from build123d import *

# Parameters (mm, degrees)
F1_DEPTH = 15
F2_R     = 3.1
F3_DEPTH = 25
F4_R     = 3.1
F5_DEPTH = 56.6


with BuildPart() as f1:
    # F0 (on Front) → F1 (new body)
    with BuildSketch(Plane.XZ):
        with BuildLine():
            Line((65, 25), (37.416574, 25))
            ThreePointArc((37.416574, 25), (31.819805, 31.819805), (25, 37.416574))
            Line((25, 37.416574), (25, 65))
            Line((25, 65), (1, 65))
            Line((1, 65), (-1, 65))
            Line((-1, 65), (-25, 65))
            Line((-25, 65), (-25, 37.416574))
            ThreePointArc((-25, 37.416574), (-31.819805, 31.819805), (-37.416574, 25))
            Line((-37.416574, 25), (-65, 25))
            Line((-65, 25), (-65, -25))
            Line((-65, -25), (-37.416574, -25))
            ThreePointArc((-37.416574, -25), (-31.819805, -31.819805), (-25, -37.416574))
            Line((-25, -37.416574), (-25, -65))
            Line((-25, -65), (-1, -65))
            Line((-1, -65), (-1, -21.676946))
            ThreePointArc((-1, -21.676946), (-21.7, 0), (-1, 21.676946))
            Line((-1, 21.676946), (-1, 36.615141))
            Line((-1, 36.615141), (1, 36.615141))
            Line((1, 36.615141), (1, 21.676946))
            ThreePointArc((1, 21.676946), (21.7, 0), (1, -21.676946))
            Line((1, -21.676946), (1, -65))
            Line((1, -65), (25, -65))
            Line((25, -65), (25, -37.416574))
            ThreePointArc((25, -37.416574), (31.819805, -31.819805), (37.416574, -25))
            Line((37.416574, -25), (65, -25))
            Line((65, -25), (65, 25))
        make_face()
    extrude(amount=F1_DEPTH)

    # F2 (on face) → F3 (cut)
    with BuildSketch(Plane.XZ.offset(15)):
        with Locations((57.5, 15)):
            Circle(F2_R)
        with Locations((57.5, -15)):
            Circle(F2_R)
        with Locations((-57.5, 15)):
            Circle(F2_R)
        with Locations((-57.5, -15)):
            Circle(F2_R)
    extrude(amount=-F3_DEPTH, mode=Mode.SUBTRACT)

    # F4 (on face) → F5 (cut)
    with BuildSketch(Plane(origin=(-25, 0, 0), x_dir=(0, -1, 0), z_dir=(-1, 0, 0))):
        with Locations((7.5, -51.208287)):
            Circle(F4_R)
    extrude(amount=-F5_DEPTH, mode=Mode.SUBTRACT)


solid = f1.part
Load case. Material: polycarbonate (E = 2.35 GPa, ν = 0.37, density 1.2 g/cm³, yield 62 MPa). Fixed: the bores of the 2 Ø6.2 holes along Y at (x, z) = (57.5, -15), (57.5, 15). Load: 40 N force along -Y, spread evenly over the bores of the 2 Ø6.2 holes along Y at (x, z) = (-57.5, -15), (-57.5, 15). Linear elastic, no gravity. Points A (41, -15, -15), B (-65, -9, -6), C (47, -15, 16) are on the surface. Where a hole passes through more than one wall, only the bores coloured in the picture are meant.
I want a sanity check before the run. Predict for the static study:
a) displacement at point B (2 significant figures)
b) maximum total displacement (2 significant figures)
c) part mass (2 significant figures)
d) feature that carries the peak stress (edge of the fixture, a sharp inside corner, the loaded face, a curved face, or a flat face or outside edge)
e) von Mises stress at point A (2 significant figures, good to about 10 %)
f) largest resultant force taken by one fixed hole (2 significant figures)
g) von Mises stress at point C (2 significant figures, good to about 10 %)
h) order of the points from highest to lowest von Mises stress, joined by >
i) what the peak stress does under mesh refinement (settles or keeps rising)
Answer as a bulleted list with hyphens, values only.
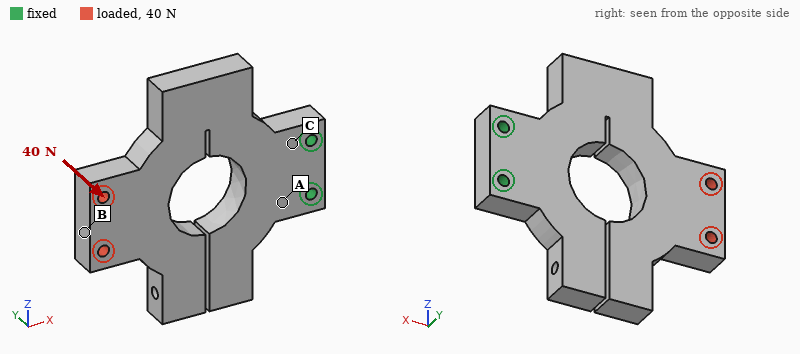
- 1.7 mm
- 1.9 mm
- 160 g
- a sharp inside corner
- 1.5 MPa
- 21 N
- 3.2 MPa
- C > A > B
- keeps rising
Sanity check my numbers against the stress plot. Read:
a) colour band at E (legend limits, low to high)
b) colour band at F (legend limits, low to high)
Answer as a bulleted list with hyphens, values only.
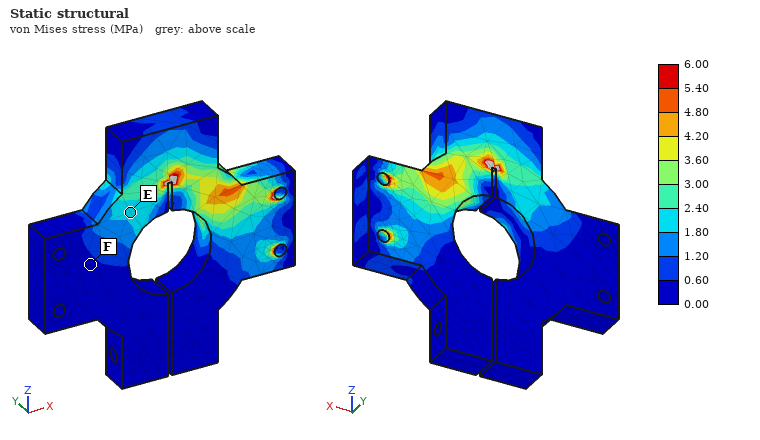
- 1.80 to 2.40 MPa
- 0.00 to 0.60 MPa
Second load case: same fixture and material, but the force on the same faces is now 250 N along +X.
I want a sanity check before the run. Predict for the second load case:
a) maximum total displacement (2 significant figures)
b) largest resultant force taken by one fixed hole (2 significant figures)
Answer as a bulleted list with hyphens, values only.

- 1.9 mm
- 130 N
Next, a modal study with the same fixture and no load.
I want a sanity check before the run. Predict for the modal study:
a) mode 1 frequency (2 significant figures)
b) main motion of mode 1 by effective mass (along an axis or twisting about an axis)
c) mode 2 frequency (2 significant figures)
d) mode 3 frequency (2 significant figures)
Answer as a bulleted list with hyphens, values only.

- 120 Hz
- along Y
- 190 Hz
- 240 Hz
